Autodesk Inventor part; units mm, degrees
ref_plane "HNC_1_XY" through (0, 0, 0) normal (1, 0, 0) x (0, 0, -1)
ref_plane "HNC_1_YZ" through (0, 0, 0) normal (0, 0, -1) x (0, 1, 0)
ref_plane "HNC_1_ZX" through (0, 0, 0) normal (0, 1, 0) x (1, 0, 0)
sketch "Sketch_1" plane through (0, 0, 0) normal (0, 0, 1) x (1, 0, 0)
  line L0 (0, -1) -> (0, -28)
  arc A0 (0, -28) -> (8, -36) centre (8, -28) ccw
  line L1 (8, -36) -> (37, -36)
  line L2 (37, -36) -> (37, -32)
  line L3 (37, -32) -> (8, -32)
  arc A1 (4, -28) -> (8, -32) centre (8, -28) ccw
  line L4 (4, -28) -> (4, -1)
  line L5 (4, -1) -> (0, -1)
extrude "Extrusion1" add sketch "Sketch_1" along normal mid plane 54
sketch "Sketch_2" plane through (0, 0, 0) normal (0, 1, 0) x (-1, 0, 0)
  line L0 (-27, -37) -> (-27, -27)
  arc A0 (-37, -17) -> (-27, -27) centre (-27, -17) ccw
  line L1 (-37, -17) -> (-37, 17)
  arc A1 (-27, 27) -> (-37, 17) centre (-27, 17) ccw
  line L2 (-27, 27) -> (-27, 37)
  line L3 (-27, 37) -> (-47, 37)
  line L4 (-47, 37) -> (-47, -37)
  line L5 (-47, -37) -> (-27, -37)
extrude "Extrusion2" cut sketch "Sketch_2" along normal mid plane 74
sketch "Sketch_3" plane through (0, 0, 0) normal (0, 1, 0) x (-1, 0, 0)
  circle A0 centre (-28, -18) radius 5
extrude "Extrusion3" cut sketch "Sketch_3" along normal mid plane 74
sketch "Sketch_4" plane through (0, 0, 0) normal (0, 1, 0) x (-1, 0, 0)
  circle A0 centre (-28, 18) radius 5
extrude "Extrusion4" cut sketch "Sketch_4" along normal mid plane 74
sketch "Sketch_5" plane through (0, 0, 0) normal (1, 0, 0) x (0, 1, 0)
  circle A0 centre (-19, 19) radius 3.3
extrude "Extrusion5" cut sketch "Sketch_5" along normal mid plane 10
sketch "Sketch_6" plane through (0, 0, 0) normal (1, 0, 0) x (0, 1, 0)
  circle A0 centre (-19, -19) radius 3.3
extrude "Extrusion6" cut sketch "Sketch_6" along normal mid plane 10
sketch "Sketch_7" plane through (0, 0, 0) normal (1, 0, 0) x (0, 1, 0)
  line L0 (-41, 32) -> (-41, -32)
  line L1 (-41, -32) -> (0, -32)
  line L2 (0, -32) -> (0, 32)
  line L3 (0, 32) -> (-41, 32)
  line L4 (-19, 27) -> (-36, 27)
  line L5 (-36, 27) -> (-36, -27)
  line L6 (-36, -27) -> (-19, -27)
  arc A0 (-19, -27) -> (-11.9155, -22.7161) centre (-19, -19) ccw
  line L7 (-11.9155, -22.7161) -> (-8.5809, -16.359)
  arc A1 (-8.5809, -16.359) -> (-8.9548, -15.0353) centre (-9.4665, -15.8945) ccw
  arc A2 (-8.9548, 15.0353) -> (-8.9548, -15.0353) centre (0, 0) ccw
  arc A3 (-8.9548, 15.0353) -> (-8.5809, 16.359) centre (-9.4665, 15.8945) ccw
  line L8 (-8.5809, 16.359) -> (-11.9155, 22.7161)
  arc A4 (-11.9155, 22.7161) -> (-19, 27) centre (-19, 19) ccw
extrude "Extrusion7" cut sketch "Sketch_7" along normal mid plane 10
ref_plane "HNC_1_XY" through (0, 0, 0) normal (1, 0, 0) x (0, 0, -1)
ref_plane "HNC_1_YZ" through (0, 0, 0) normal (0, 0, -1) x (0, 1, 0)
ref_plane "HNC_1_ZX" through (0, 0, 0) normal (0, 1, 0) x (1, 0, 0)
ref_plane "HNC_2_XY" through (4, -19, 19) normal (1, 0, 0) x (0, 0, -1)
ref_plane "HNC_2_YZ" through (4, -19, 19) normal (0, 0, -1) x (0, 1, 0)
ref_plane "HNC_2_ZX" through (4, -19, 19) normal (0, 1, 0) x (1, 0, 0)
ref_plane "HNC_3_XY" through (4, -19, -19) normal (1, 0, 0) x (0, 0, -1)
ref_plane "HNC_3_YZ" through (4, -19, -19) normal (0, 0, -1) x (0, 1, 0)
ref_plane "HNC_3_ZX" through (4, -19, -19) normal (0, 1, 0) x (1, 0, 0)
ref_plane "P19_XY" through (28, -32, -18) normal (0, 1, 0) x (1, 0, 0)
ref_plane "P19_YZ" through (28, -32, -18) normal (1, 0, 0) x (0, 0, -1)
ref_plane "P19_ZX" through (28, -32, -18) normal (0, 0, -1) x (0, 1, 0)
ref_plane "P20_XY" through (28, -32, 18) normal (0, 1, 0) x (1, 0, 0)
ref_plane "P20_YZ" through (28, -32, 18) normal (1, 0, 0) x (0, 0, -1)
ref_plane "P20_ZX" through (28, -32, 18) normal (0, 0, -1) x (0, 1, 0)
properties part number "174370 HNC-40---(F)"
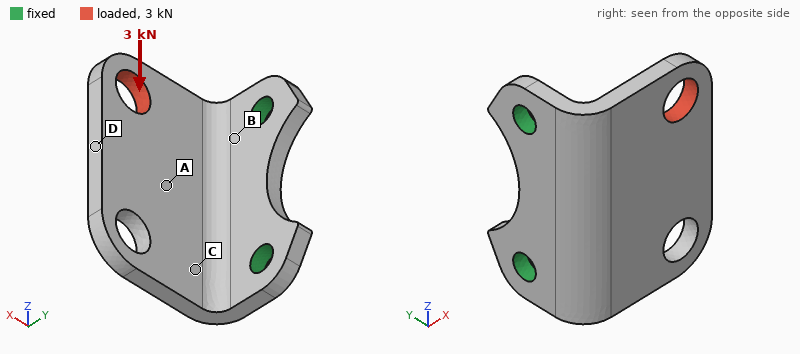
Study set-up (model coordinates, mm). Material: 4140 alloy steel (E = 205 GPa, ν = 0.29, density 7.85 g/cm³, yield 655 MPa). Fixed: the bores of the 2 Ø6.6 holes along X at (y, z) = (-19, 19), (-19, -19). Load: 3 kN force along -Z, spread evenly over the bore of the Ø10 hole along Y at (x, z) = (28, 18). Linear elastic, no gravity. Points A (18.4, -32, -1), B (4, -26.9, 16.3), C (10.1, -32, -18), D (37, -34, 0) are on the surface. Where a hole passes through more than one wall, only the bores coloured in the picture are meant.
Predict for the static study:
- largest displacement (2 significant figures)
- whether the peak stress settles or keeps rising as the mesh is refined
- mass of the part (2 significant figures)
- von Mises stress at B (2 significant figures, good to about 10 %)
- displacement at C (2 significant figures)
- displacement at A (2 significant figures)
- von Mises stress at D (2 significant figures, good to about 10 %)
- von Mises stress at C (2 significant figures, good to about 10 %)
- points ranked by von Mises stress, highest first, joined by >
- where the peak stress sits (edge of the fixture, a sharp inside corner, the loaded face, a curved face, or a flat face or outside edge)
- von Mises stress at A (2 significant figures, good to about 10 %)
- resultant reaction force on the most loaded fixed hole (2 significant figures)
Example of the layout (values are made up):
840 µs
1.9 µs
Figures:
0.12 mm
keeps rising
81 g
160 MPa
0.045 mm
0.042 mm
32 MPa
120 MPa
B > C > A > D
edge of the fixture
69 MPa
2.6 kN
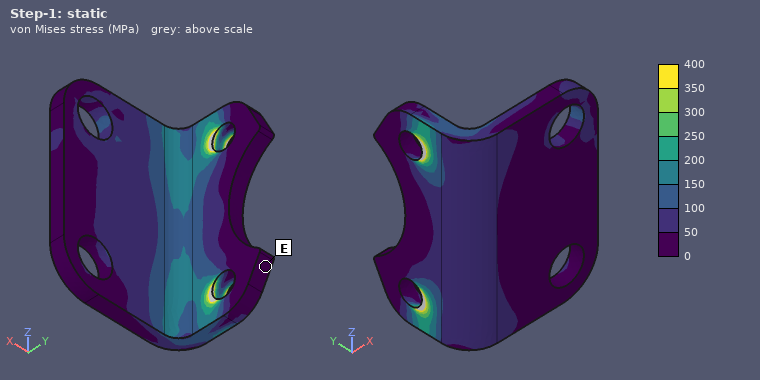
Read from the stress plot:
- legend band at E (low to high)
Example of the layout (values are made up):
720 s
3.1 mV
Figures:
0 to 50 MPa
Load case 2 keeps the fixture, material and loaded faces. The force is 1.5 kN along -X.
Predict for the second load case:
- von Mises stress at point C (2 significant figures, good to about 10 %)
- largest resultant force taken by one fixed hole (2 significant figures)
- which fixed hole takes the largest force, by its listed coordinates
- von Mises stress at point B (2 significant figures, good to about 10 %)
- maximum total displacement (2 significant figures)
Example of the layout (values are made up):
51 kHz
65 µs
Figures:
26 MPa
1.4 kN
(-19, 19)
130 MPa
0.13 mm
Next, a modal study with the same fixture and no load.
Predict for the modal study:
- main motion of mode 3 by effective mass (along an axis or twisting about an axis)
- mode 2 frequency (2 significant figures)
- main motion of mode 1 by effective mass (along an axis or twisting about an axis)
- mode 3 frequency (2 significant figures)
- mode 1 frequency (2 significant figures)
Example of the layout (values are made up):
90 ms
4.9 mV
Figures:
along X
4100 Hz
along Y
6900 Hz
1900 Hz
